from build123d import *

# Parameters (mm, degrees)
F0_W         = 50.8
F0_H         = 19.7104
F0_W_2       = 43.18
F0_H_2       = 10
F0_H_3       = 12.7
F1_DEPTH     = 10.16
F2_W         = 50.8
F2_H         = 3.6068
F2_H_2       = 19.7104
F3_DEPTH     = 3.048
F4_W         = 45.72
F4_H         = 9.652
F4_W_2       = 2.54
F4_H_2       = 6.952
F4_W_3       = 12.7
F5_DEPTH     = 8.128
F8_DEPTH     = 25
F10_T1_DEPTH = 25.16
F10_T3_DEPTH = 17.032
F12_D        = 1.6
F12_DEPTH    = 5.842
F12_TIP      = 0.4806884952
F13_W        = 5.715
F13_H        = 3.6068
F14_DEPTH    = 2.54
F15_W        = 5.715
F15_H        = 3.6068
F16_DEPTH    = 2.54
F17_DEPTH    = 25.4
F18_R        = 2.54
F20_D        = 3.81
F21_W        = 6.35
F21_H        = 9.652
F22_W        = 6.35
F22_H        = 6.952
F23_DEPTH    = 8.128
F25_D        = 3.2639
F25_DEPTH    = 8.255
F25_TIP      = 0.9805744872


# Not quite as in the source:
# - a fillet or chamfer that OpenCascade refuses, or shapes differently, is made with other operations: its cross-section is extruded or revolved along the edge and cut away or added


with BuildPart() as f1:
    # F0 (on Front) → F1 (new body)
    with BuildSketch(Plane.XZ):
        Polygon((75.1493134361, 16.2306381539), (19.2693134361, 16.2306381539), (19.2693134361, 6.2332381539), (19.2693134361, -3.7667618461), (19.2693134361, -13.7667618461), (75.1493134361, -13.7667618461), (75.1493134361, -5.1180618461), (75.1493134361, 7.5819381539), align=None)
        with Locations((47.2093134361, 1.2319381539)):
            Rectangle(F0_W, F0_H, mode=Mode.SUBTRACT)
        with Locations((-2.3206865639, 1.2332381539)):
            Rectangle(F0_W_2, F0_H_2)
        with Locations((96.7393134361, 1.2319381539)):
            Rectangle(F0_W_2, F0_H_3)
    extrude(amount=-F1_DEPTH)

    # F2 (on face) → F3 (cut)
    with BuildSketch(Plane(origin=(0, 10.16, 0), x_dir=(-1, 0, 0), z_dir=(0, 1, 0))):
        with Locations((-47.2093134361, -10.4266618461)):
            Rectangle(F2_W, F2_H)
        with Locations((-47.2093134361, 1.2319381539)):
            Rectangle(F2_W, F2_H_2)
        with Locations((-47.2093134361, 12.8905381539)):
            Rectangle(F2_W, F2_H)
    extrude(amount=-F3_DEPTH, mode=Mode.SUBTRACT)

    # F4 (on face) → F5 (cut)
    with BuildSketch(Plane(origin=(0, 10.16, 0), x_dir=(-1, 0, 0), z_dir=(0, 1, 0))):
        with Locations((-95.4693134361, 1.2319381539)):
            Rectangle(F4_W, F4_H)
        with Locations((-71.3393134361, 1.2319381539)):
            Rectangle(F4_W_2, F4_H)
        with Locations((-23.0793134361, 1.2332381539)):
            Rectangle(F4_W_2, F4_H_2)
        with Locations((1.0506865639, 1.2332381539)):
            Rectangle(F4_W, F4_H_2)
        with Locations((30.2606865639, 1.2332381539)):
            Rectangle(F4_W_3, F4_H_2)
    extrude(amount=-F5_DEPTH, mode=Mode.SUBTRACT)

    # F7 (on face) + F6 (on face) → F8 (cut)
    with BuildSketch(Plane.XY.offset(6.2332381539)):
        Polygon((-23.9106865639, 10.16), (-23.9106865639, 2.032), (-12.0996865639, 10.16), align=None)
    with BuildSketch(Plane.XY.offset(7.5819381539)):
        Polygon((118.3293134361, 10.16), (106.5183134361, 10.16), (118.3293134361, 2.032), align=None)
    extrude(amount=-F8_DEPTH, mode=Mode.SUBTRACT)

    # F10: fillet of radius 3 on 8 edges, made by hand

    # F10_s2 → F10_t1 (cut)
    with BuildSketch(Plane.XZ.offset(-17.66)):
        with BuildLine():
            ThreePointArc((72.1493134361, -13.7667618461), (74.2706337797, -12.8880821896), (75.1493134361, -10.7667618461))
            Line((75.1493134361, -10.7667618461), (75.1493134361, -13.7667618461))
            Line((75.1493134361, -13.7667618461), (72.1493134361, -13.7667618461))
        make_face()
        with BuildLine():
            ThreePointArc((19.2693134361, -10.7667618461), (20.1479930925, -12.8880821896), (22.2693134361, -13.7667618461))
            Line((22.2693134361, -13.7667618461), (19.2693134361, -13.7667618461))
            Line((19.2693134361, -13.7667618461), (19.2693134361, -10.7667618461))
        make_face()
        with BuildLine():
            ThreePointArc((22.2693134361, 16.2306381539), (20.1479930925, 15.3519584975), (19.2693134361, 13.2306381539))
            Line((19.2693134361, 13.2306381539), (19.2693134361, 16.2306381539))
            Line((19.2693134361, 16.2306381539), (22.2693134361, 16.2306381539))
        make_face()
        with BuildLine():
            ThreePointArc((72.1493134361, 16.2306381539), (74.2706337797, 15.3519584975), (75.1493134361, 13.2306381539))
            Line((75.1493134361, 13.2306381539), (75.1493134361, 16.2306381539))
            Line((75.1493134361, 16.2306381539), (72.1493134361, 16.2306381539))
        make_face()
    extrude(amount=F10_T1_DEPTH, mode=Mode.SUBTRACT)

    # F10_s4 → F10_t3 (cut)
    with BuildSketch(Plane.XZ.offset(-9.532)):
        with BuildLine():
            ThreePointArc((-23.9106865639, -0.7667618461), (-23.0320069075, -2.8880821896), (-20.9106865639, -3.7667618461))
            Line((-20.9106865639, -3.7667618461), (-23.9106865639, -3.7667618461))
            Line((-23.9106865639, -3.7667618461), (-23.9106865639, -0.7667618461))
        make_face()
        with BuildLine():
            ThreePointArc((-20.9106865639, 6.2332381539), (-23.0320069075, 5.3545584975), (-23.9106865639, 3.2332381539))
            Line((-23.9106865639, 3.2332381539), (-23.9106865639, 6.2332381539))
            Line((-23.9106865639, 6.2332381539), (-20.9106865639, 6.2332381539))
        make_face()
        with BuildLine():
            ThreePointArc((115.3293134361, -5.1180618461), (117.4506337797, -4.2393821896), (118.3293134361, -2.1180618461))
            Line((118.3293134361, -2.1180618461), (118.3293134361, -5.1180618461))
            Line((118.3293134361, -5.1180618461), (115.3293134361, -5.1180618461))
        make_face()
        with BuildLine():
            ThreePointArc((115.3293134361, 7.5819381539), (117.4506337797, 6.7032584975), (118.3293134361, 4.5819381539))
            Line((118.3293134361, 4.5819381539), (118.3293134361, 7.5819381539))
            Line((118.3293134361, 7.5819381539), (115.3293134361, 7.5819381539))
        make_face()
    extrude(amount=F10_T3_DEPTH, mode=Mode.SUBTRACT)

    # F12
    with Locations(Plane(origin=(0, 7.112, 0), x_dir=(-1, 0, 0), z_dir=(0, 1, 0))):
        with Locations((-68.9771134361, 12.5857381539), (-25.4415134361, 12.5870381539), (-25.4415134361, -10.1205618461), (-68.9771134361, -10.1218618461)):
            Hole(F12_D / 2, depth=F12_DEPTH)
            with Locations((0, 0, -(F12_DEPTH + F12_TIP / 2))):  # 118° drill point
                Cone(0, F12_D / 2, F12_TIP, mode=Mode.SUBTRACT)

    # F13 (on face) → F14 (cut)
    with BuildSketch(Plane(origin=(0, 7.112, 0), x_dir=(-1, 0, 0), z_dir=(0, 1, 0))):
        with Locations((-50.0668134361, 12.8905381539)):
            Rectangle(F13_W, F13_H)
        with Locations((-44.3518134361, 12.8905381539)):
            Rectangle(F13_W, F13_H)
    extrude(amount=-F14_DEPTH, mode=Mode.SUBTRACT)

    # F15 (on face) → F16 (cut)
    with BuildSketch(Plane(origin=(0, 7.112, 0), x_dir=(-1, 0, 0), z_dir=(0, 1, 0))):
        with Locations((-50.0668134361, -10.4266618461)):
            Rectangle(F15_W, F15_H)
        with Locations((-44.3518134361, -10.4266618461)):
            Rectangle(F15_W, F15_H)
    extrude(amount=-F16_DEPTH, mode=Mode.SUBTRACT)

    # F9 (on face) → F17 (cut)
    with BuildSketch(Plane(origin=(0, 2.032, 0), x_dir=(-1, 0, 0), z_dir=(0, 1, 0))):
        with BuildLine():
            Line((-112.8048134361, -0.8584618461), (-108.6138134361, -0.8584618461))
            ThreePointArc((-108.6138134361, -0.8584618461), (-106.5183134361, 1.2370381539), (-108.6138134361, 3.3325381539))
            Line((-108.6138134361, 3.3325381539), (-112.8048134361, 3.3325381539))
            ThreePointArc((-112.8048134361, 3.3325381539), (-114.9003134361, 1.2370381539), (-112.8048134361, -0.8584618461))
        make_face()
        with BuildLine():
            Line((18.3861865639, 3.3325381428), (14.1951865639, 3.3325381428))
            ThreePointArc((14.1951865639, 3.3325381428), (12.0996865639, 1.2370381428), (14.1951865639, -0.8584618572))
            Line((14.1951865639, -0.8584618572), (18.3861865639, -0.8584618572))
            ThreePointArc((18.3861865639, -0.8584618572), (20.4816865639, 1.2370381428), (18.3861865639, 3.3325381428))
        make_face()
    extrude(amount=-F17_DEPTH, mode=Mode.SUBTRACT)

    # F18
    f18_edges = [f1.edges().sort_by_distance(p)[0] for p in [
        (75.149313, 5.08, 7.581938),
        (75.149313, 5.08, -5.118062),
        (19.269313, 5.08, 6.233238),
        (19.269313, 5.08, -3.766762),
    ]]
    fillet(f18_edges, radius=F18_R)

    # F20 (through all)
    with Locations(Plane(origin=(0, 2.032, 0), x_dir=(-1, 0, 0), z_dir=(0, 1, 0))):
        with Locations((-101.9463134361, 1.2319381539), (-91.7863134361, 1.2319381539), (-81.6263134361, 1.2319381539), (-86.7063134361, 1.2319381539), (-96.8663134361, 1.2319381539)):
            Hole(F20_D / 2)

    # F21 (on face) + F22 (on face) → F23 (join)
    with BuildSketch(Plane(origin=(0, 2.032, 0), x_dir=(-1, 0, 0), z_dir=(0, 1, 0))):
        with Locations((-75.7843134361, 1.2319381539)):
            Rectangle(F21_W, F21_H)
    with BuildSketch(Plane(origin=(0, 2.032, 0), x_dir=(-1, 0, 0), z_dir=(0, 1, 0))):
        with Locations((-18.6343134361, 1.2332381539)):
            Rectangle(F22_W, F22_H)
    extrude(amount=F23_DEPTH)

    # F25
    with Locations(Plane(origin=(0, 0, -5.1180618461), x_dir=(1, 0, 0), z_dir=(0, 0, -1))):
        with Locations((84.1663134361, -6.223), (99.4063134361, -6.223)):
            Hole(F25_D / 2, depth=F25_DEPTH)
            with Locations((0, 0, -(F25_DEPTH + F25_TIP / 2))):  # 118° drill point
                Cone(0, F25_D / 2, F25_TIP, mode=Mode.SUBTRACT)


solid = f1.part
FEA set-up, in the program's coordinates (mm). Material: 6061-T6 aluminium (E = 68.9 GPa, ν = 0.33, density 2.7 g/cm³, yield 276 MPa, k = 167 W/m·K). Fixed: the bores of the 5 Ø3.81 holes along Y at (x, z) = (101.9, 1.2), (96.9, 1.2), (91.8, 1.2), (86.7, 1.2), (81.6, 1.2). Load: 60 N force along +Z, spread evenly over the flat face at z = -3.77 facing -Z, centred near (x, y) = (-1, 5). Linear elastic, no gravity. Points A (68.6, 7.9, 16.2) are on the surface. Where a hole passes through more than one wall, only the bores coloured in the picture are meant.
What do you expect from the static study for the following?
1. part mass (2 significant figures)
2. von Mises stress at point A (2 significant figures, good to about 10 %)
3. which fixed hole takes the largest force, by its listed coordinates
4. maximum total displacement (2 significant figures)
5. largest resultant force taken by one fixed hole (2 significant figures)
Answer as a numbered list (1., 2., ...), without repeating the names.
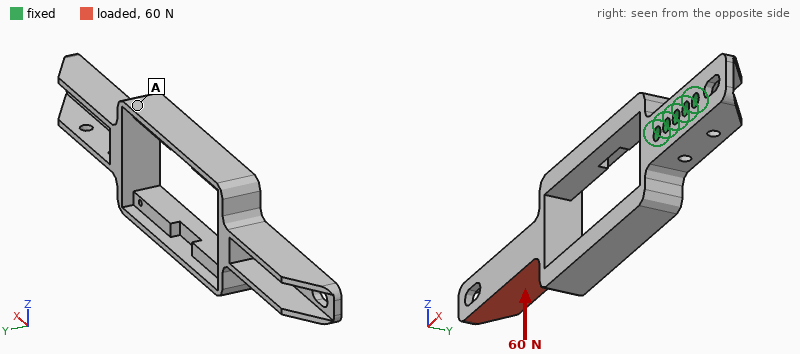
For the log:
1. 26 g
2. 15 MPa
3. (81.6, 1.2)
4. 0.53 mm
5. 300 N
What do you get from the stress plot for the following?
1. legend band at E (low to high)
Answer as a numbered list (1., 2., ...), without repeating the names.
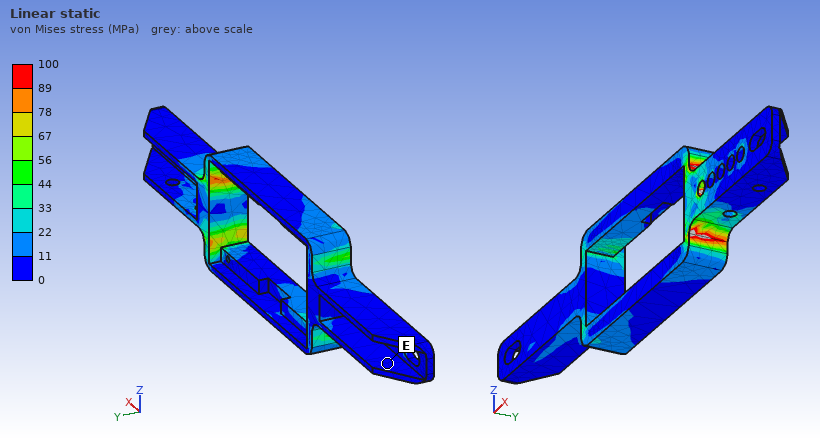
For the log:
1. 0 to 11 MPa
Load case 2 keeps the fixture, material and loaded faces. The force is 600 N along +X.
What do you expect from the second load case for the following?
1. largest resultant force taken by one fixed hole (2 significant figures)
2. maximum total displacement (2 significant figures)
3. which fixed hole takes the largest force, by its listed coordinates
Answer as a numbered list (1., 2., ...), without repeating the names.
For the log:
1. 320 N
2. 0.37 mm
3. (81.6, 1.2)
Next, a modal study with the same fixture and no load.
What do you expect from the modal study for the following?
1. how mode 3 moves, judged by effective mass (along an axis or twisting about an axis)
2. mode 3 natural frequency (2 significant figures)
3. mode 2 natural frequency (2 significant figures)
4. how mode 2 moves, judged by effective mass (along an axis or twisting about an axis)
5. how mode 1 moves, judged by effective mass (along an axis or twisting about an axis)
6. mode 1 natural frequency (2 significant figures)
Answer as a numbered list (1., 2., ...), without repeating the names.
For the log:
1. twisting about X
2. 2000 Hz
3. 590 Hz
4. along Z
5. along Y
6. 510 Hz
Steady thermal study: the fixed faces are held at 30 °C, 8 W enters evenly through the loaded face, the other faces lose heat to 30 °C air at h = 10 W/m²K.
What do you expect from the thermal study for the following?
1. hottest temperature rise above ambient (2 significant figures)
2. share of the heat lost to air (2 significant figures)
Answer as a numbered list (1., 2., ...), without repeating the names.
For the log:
1. 61 K
2. 25 %
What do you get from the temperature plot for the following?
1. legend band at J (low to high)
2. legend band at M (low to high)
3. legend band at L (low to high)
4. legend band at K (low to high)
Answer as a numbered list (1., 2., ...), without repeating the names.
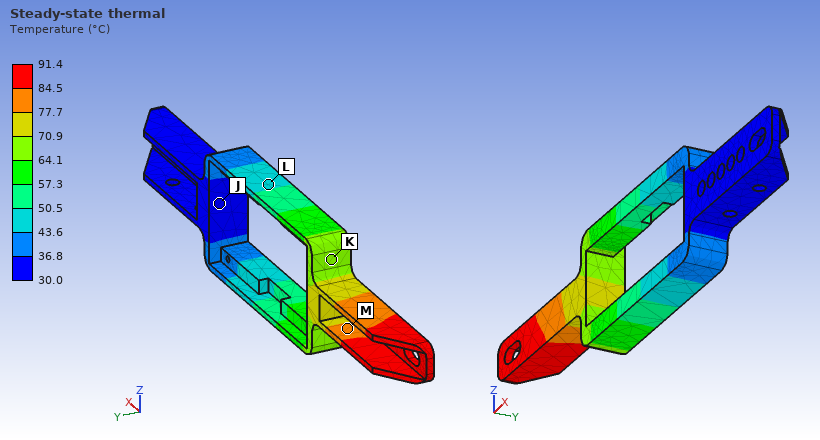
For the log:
1. 30.0 to 36.8 °C
2. 77.7 to 84.5 °C
3. 43.6 to 50.5 °C
4. 64.1 to 70.9 °C
